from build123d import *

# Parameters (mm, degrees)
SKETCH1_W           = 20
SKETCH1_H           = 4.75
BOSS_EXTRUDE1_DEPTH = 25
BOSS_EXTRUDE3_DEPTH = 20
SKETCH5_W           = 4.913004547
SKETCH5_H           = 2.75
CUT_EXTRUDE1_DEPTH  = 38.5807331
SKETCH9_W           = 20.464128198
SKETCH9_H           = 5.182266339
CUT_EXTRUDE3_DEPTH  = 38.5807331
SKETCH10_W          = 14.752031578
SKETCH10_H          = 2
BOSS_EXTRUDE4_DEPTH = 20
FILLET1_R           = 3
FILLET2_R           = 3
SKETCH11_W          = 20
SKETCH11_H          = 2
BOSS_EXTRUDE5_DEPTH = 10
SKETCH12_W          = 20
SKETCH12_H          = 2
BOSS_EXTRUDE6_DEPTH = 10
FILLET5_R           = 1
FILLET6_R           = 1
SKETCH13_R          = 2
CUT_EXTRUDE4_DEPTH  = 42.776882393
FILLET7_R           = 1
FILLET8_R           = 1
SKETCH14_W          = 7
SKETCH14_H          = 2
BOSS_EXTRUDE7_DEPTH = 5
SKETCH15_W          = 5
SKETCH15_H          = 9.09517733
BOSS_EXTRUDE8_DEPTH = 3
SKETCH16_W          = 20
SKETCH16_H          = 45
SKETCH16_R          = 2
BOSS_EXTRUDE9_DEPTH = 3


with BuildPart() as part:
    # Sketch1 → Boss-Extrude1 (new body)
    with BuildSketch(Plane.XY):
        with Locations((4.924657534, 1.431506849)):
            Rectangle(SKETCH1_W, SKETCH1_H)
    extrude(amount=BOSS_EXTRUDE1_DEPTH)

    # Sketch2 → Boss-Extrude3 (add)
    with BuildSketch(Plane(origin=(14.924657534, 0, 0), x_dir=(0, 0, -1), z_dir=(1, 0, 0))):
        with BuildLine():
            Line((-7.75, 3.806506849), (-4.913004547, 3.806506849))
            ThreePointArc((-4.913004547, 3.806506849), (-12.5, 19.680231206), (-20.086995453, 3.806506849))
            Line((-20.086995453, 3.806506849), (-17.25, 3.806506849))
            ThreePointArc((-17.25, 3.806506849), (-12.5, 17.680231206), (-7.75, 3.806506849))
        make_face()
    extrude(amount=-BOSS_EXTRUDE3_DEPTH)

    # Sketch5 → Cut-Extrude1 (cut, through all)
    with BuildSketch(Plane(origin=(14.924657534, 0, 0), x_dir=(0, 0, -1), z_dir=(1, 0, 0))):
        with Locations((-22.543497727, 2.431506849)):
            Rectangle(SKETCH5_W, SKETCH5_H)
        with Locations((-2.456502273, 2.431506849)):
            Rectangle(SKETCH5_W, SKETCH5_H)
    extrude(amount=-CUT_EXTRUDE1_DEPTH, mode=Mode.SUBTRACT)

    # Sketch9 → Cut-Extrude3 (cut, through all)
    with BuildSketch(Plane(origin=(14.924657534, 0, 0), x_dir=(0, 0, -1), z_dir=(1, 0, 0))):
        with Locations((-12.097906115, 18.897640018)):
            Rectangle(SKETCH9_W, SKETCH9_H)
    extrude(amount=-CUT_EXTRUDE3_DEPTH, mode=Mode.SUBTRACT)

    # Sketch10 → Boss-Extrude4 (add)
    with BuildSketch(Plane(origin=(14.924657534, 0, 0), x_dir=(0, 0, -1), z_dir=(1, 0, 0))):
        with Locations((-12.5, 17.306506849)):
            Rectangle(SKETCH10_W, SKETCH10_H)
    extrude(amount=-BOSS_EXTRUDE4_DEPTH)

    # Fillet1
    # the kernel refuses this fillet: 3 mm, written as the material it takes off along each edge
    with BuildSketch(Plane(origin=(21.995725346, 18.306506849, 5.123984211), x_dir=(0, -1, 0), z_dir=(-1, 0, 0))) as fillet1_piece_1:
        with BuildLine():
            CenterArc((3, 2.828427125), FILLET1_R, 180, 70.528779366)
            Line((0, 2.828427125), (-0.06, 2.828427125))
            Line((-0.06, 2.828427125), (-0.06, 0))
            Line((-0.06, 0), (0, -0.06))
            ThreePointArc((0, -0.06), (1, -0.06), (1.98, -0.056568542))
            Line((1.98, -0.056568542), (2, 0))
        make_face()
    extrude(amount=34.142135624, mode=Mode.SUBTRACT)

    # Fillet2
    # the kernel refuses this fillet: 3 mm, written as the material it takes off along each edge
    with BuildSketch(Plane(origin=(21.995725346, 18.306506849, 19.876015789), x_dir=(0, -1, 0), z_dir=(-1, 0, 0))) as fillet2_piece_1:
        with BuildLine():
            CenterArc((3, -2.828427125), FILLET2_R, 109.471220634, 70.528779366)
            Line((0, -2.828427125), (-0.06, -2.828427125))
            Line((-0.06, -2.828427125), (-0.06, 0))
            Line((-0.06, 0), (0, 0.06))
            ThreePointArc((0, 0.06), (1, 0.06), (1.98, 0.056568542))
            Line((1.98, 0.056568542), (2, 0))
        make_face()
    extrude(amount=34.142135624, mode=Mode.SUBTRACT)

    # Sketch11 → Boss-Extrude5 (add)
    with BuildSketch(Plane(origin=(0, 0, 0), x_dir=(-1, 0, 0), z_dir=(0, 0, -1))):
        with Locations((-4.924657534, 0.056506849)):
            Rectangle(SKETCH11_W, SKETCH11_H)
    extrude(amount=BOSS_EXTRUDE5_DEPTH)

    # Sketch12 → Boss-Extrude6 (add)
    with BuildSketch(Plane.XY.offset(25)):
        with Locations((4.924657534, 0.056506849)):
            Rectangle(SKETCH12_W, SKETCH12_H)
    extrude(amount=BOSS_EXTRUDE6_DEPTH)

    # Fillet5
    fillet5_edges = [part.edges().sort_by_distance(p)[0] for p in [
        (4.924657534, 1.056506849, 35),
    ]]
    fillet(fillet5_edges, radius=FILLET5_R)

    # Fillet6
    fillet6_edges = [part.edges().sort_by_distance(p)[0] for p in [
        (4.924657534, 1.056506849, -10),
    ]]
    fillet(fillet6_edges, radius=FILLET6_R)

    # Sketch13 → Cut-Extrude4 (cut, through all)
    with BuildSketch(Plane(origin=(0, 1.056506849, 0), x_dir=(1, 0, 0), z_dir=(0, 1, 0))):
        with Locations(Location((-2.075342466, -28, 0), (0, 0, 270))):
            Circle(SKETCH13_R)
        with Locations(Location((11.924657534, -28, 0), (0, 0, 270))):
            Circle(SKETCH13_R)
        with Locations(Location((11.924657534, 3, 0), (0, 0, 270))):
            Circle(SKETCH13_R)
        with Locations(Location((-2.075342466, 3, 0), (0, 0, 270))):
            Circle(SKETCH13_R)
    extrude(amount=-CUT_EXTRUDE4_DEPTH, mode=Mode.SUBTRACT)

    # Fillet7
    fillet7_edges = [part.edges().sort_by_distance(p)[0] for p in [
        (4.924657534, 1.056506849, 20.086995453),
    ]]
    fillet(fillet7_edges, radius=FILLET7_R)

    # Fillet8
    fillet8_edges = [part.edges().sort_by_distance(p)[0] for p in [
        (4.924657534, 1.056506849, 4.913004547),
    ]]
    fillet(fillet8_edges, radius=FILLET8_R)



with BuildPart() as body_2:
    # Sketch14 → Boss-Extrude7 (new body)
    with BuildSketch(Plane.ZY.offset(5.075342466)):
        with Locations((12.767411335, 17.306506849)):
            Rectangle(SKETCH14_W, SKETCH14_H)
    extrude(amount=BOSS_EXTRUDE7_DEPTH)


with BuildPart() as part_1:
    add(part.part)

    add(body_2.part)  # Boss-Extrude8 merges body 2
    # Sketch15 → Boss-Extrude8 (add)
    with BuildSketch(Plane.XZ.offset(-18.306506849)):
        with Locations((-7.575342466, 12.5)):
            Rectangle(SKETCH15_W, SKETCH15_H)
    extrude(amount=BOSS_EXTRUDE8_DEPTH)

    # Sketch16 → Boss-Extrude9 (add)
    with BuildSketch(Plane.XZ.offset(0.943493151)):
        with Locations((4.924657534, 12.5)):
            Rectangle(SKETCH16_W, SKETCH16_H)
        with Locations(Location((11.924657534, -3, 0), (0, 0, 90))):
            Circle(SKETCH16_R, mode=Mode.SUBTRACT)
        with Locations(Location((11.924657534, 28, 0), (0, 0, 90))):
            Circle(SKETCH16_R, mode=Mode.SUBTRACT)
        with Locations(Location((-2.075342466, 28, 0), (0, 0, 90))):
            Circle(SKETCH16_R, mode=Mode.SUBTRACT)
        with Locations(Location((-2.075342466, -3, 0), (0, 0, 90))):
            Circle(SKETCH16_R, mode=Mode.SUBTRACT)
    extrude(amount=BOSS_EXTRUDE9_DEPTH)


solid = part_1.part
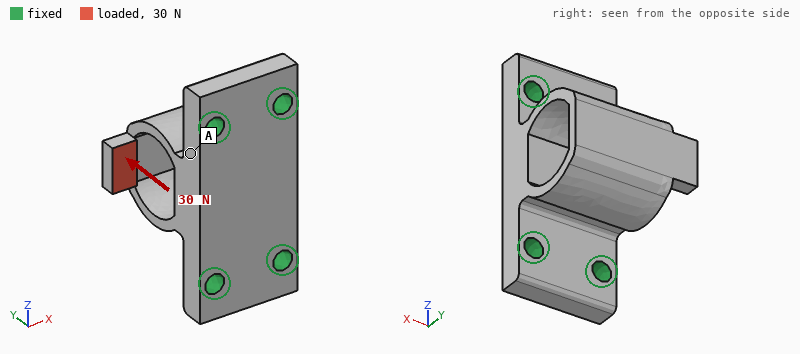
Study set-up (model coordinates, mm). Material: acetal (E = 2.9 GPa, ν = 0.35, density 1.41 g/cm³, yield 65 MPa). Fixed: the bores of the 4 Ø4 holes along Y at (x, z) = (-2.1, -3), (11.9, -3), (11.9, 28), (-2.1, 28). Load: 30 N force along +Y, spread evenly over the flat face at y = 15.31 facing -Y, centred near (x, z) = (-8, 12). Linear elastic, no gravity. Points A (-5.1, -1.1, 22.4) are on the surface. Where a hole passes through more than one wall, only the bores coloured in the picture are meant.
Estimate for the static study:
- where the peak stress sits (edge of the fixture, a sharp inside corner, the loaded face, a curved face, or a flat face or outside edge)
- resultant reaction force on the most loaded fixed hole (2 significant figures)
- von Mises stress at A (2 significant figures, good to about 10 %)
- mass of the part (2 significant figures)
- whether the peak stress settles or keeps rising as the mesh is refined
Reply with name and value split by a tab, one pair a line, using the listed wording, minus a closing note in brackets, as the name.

where the peak stress sits	a sharp inside corner
resultant reaction force on the most loaded fixed hole	20 N
von Mises stress at A	2.1 MPa
mass of the part	9.7 g
whether the peak stress settles or keeps rising as the mesh is refined	keeps rising
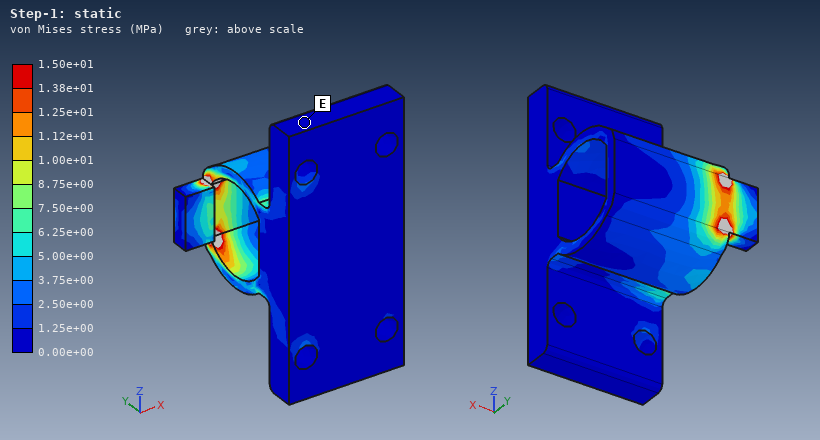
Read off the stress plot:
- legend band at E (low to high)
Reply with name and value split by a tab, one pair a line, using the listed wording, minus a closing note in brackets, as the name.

legend band at E	0.00e+00 to 1.25e+00 MPa
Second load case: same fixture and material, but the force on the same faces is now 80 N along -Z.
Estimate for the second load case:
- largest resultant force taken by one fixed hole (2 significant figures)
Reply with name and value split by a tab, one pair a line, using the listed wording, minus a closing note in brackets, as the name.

largest resultant force taken by one fixed hole	49 N
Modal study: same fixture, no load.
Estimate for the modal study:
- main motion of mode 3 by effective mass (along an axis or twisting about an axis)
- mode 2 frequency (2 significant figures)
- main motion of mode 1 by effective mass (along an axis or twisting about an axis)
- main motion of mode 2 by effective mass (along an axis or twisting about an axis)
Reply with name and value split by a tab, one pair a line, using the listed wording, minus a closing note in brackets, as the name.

main motion of mode 3 by effective mass	along Y
mode 2 frequency	3000 Hz
main motion of mode 1 by effective mass	along Z
main motion of mode 2 by effective mass	along X
